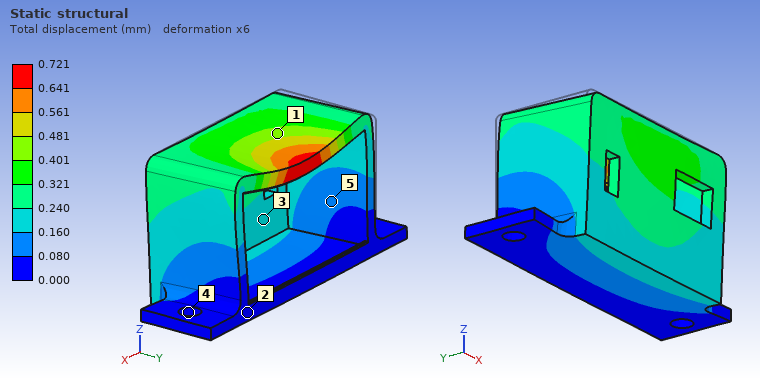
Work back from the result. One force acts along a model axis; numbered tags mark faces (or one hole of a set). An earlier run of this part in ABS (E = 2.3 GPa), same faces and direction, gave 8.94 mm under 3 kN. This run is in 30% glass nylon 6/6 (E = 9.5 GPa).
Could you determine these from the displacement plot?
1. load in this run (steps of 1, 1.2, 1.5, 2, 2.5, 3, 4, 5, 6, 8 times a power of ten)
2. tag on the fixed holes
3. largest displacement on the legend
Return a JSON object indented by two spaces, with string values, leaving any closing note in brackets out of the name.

{
  "load in this run": "1 kN",
  "tag on the fixed holes": "4",
  "largest displacement on the legend": "0.721 mm"
}
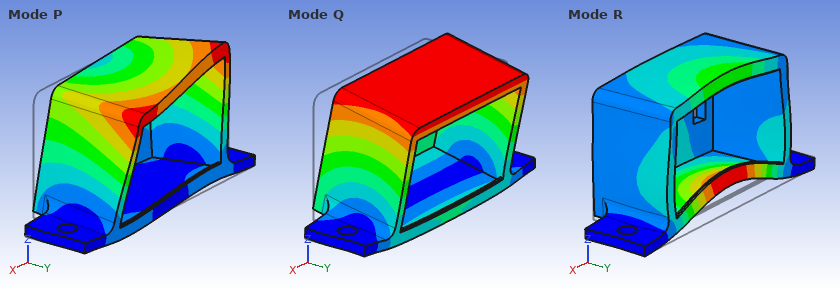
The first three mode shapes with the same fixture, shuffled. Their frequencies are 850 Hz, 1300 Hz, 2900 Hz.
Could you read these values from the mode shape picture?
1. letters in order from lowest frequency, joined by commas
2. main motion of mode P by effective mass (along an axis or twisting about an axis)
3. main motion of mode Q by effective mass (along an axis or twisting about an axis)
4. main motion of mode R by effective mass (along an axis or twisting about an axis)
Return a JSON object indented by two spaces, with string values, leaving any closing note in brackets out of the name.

{
  "letters in order from lowest frequency, joined by commas": "Q, P, R",
  "main motion of mode P by effective mass": "along X",
  "main motion of mode Q by effective mass": "along Y",
  "main motion of mode R by effective mass": "along Z"
}
